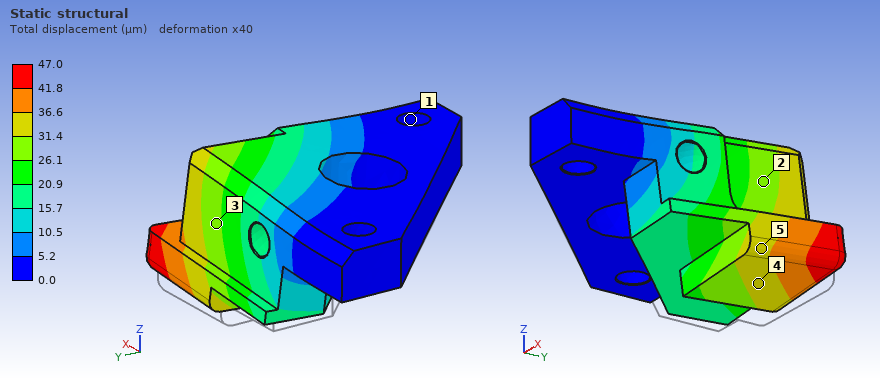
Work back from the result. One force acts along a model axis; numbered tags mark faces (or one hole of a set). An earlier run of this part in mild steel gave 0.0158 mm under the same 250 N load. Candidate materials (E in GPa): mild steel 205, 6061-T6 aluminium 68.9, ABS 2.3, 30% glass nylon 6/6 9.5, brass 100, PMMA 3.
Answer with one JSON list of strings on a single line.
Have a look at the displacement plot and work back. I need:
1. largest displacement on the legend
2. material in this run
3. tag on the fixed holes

["47.0 µm", "6061-T6 aluminium", "1"]
